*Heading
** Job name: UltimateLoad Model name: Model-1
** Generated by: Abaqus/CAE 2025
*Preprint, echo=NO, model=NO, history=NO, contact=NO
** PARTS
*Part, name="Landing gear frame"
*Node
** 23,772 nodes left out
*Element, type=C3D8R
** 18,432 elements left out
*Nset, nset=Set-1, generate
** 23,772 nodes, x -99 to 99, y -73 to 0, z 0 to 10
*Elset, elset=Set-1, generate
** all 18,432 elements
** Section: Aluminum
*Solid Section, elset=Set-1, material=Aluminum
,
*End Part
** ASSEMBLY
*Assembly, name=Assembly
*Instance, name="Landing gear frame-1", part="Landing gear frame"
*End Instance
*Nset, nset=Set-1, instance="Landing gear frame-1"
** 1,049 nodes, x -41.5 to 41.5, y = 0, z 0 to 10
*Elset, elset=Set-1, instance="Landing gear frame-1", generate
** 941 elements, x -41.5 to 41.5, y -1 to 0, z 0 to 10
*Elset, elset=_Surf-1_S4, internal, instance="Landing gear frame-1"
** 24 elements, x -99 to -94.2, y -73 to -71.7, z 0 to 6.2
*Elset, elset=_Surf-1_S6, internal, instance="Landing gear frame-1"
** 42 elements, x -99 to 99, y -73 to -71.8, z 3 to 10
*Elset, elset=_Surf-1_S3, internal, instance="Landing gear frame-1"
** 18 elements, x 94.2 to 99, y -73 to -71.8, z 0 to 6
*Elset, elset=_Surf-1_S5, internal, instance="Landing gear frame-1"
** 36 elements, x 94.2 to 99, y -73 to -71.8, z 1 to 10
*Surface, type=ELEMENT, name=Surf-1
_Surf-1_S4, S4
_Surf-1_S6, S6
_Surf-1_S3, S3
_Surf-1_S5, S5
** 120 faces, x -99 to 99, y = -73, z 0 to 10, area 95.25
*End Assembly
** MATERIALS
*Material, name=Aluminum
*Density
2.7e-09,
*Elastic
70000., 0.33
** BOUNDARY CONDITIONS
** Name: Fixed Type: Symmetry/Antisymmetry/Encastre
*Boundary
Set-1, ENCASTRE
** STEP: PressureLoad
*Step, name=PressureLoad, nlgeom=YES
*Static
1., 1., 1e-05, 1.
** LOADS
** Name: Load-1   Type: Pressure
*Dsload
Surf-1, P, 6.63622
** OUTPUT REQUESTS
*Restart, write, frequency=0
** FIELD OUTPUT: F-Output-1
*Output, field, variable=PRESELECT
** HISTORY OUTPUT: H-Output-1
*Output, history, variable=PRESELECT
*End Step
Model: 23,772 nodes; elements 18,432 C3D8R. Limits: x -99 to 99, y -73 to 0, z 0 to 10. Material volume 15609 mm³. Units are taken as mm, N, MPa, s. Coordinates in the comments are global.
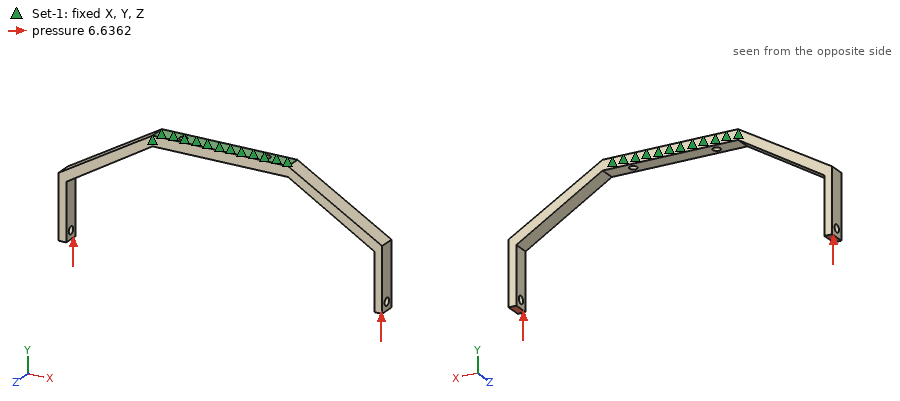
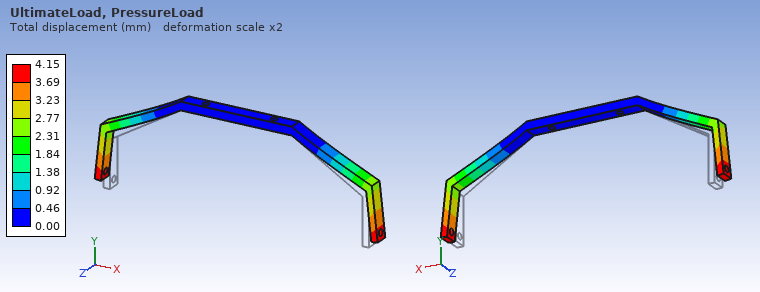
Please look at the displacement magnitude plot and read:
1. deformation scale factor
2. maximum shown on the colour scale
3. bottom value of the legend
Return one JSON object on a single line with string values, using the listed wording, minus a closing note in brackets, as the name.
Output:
{"deformation scale factor": "2", "maximum shown on the colour scale": "4.15 mm", "bottom value of the legend": "0.00 mm"}
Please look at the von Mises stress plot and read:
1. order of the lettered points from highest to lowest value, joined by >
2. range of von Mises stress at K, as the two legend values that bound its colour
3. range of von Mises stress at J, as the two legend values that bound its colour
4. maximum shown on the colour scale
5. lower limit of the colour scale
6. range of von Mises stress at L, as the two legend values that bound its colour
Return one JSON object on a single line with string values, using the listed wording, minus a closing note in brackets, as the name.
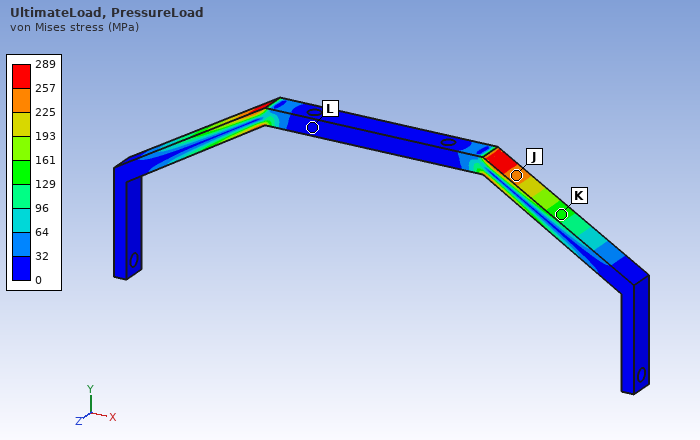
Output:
{"order of the lettered points from highest to lowest value, joined by >": "J > K > L", "range of von Mises stress at K, as the two legend values that bound its colour": "129 to 161 MPa", "range of von Mises stress at J, as the two legend values that bound its colour": "225 to 257 MPa", "maximum shown on the colour scale": "289 MPa", "lower limit of the colour scale": "0 MPa", "range of von Mises stress at L, as the two legend values that bound its colour": "0 to 32 MPa"}
